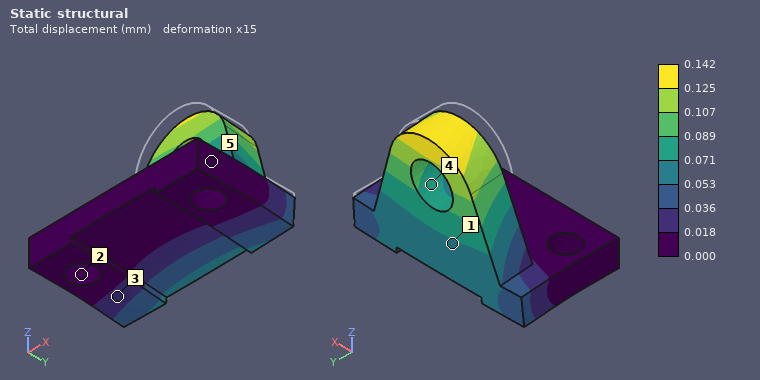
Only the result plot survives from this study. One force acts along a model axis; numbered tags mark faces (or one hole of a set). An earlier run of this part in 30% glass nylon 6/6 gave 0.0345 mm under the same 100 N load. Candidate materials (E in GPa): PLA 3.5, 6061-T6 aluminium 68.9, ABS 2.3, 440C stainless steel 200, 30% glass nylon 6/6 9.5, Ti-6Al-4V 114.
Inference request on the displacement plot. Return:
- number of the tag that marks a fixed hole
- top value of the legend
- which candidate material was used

2
0.142 mm
ABS
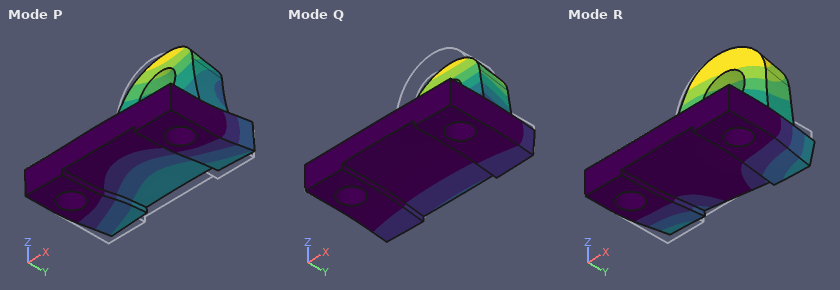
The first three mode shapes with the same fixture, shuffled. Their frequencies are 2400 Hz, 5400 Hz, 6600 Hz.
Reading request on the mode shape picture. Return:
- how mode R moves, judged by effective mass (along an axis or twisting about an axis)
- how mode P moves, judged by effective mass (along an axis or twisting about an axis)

along X
along Z
